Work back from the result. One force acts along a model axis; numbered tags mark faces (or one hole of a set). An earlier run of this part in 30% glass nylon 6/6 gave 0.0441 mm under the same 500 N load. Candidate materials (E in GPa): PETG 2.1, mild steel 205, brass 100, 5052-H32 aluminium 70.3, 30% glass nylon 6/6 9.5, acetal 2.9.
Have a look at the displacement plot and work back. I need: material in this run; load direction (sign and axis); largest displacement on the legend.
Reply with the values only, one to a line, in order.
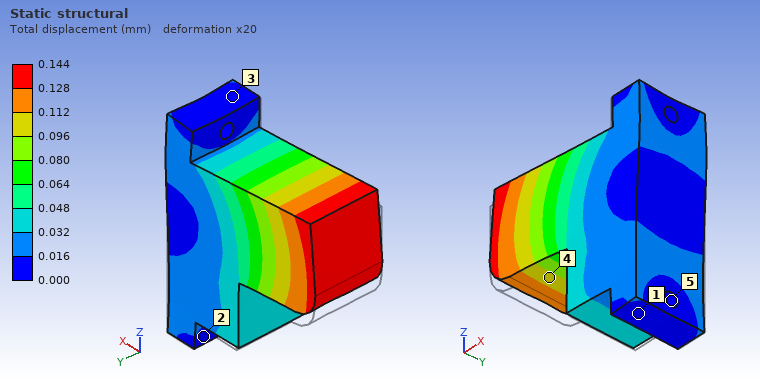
acetal
+Z
0.144 mm
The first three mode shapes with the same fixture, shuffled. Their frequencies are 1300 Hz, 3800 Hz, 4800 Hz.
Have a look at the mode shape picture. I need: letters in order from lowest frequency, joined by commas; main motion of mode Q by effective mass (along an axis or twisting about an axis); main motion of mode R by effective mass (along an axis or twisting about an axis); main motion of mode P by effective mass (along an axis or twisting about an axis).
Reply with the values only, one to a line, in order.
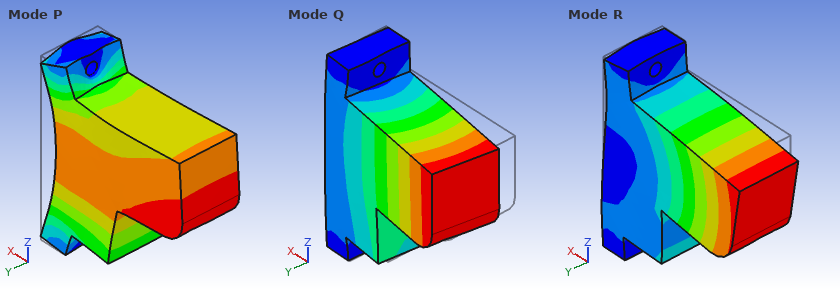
Q, R, P
along Y
along Z
along X
